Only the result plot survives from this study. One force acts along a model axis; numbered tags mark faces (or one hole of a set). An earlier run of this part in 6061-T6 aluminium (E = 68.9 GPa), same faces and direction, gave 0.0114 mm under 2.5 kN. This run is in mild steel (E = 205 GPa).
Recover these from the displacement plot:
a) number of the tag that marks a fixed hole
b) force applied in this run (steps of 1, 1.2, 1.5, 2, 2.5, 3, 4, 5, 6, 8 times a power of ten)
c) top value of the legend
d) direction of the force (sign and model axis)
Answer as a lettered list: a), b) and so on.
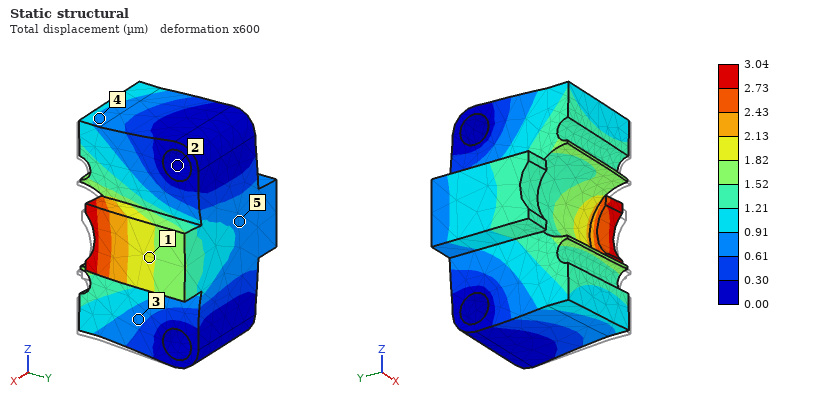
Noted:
a) 2
b) 2 kN
c) 3.04 µm
d) -X
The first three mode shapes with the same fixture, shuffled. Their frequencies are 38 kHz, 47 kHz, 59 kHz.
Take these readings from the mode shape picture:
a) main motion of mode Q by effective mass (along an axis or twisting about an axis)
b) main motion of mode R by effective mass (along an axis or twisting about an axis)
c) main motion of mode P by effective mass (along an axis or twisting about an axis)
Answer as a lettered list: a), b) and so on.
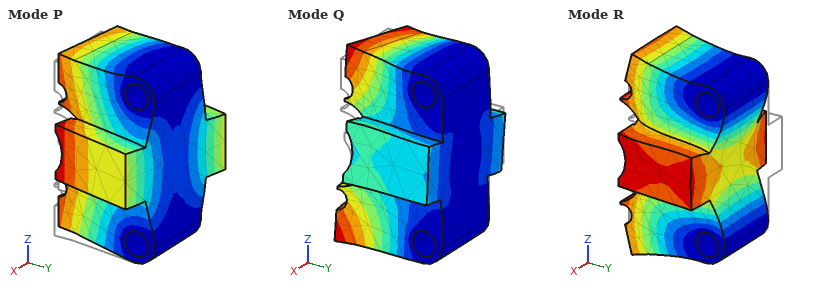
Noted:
a) twisting about Y
b) along Y
c) along X
